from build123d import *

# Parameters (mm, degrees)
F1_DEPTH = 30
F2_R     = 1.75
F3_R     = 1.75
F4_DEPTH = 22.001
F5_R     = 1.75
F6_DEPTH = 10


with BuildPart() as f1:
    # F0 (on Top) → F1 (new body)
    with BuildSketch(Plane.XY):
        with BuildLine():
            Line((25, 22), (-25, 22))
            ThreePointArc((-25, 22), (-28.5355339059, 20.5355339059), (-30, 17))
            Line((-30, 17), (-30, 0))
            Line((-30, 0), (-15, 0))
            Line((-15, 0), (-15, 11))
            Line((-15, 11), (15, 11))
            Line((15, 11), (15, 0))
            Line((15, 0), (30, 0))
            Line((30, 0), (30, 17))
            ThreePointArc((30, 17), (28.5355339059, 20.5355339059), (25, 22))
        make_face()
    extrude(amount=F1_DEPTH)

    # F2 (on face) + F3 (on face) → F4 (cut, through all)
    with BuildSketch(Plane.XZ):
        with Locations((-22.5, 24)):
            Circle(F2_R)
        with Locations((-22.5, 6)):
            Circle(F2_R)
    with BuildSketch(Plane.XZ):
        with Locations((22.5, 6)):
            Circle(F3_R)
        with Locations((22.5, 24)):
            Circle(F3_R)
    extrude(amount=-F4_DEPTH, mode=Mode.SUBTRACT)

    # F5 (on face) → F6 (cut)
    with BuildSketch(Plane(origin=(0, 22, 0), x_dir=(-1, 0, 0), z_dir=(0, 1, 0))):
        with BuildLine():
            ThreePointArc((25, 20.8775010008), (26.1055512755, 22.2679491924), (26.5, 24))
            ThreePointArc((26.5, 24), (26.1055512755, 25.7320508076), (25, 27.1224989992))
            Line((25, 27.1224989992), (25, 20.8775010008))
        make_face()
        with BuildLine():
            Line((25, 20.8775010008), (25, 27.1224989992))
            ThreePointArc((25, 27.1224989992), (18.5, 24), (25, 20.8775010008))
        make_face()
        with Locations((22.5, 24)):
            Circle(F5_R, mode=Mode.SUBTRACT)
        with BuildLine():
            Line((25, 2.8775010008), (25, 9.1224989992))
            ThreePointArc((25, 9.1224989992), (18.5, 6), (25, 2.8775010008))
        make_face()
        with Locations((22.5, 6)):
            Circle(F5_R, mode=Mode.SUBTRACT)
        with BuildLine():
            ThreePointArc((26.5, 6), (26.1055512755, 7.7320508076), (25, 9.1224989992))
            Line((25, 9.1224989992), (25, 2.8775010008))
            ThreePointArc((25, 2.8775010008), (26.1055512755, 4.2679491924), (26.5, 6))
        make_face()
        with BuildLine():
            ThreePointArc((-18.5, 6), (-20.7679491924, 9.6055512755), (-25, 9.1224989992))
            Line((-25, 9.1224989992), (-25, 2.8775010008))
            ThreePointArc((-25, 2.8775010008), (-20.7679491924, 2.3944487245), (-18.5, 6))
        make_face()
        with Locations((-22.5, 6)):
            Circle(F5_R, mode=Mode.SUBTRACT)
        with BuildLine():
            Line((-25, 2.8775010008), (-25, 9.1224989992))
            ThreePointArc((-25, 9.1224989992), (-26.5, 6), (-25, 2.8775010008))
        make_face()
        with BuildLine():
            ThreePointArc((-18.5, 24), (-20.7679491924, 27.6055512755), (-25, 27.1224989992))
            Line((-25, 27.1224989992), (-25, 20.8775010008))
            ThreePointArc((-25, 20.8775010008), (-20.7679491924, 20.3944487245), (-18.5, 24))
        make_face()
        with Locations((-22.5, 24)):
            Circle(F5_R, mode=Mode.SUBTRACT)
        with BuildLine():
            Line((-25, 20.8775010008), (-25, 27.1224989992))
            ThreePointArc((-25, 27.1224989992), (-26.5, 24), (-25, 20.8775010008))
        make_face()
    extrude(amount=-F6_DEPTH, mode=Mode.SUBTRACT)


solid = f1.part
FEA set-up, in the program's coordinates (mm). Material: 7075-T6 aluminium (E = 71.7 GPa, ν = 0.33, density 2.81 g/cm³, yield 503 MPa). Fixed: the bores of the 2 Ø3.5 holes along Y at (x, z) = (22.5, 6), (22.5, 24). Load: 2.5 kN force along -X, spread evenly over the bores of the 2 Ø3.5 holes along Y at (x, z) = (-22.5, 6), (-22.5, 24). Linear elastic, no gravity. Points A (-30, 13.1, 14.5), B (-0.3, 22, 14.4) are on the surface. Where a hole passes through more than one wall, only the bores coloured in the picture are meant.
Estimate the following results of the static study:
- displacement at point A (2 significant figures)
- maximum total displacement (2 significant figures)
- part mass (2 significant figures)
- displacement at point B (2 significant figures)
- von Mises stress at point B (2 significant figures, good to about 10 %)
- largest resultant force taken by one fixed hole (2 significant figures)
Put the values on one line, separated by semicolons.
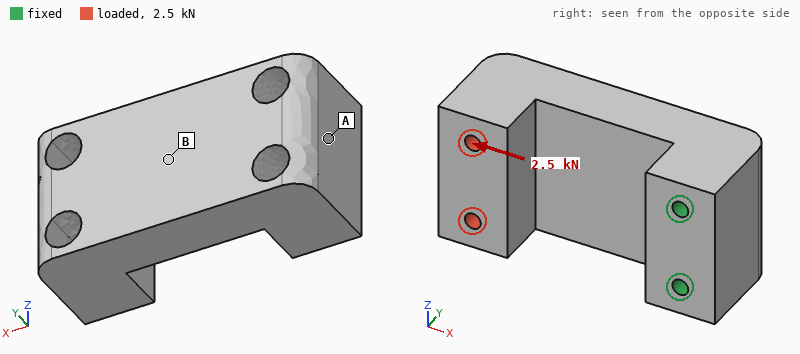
0.14 mm; 0.16 mm; 76 g; 0.030 mm; 34 MPa; 1.3 kN
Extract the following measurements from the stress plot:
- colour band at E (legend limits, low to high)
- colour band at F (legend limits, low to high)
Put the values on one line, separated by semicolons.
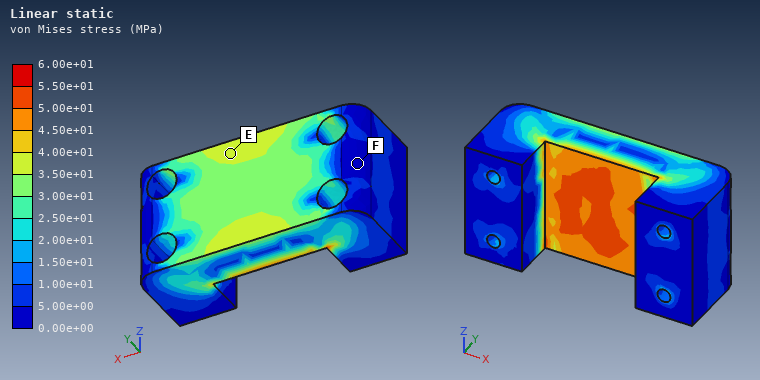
3.50e+01 to 4.00e+01 MPa; 0.00e+00 to 5.00e+00 MPa
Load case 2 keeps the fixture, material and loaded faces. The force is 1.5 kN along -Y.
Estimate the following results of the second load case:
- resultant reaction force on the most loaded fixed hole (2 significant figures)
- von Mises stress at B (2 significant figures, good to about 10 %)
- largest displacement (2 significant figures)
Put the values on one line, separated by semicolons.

880 N; 53 MPa; 0.35 mm
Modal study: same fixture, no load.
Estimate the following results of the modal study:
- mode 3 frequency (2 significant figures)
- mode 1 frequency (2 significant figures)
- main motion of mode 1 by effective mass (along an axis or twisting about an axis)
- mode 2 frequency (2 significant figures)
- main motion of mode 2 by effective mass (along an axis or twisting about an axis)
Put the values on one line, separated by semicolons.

8100 Hz; 2100 Hz; along Y; 4000 Hz; along Z
